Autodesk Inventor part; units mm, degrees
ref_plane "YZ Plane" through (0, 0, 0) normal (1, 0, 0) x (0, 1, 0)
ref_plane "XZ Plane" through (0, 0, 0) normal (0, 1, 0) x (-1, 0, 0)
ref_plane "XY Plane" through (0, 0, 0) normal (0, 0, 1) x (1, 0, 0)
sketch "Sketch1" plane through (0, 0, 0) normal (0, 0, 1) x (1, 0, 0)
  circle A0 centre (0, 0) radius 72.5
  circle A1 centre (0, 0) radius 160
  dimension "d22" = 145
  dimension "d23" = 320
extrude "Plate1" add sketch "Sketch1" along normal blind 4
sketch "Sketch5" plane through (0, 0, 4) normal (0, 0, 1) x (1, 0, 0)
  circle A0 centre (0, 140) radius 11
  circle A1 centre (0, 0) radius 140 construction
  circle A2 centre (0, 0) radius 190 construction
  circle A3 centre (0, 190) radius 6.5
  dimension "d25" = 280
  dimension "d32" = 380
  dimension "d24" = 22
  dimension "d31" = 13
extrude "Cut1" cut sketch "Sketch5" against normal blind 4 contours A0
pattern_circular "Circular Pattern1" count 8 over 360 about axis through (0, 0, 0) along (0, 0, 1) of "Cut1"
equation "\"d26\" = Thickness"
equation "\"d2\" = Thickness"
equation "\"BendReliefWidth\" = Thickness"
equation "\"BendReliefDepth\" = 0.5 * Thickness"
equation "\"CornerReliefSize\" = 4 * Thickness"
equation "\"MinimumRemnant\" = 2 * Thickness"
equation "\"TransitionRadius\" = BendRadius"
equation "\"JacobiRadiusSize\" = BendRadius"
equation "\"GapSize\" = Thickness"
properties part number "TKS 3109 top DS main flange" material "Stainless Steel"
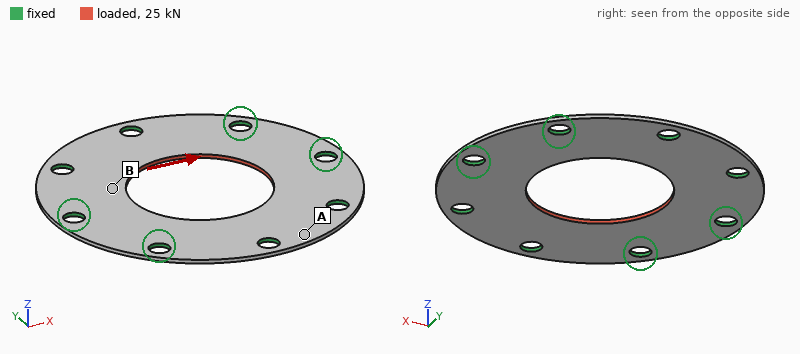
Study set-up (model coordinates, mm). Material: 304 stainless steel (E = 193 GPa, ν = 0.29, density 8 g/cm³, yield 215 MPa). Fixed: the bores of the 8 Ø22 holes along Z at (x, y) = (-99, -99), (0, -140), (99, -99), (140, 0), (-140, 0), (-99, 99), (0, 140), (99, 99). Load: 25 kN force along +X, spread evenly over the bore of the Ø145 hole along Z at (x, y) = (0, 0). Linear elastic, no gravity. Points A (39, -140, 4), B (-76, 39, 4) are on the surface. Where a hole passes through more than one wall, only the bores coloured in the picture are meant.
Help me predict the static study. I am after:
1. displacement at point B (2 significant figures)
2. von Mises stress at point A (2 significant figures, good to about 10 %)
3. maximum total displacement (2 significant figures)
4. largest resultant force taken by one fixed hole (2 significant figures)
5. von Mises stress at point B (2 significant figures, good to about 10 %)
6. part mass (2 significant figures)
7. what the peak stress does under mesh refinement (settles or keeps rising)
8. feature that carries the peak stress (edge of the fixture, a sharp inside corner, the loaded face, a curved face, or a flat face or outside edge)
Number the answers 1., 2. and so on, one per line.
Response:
1. 5.2 µm
2. 2.7 MPa
3. 6.7 µm
4. 4.6 kN
5. 12 MPa
6. 1.9 kg
7. keeps rising
8. edge of the fixture
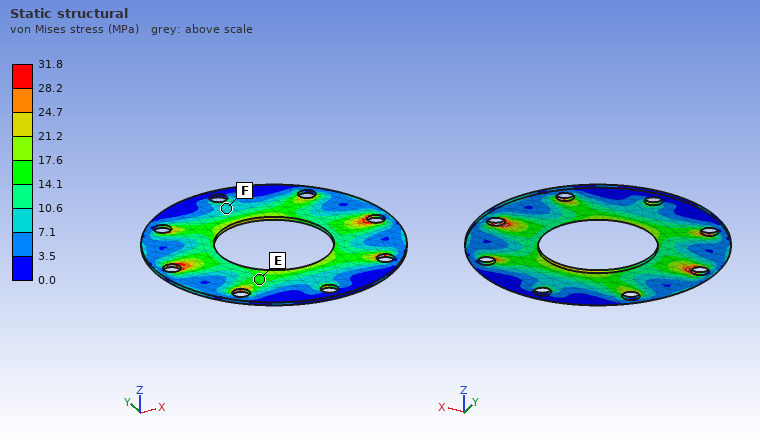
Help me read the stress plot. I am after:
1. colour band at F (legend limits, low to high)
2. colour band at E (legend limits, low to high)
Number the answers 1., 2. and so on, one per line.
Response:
1. 7.1 to 10.6 MPa
2. 14.1 to 17.6 MPa
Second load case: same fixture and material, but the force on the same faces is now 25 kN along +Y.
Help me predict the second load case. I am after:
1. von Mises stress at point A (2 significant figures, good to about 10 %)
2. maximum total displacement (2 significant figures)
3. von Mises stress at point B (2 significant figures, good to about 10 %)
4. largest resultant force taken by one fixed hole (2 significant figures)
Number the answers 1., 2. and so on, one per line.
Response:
1. 5.1 MPa
2. 6.7 µm
3. 17 MPa
4. 4.6 kN
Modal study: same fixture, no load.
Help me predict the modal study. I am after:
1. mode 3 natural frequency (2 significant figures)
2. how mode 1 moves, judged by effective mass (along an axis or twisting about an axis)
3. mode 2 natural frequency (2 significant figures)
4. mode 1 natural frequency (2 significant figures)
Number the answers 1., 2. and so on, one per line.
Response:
1. 1100 Hz
2. along Z
3. 1100 Hz
4. 950 Hz
